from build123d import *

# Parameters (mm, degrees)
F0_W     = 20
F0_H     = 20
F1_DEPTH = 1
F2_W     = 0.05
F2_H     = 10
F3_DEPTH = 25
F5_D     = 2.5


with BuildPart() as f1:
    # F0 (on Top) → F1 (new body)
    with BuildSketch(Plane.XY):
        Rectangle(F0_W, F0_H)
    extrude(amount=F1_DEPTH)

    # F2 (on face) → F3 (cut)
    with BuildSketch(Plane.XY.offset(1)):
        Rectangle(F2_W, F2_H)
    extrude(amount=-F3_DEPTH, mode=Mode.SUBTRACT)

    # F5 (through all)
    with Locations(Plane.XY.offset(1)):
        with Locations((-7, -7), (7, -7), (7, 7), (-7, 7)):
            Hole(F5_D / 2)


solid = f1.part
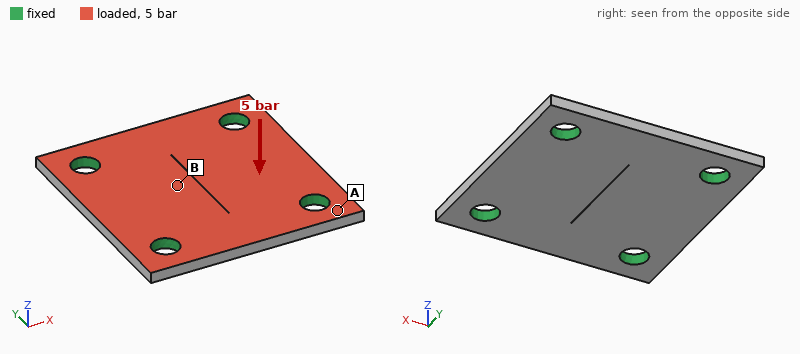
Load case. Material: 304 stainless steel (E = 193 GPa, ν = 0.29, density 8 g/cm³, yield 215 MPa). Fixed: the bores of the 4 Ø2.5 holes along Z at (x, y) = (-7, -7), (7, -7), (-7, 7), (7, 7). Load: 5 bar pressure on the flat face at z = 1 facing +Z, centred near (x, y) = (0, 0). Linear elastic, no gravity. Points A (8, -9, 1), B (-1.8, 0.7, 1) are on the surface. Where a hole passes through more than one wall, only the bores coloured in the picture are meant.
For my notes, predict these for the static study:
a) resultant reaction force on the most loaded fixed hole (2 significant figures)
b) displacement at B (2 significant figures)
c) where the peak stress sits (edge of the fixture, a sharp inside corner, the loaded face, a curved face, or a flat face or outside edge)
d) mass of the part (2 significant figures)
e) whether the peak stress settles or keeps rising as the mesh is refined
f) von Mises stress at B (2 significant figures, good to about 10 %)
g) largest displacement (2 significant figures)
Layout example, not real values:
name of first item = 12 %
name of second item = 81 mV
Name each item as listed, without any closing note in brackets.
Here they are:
resultant reaction force on the most loaded fixed hole = 47 N
displacement at B = 5.8 µm
where the peak stress sits = a sharp inside corner
mass of the part = 3.0 g
whether the peak stress settles or keeps rising as the mesh is refined = keeps rising
von Mises stress at B = 21 MPa
largest displacement = 7.4 µm
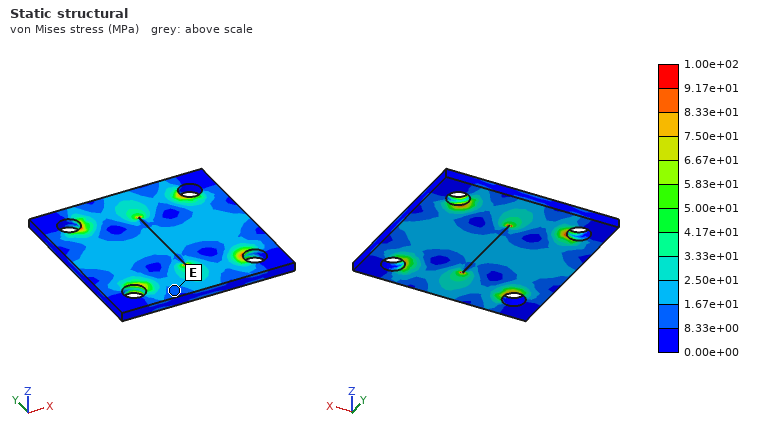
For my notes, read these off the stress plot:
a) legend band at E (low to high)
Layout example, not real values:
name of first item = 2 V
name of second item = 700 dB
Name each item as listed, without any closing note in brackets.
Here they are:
legend band at E = 8.33e+00 to 1.67e+01 MPa
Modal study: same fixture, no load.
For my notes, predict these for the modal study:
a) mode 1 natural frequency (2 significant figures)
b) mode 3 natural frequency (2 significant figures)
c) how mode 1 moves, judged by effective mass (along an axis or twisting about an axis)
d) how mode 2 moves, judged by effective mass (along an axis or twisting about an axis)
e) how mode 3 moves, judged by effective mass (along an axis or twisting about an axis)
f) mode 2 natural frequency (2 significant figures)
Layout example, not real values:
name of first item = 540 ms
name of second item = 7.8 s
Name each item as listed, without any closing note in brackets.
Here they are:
mode 1 natural frequency = 20 kHz
mode 3 natural frequency = 33 kHz
how mode 1 moves, judged by effective mass = along Z
how mode 2 moves, judged by effective mass = twisting about Y
how mode 3 moves, judged by effective mass = twisting about X
mode 2 natural frequency = 31 kHz
